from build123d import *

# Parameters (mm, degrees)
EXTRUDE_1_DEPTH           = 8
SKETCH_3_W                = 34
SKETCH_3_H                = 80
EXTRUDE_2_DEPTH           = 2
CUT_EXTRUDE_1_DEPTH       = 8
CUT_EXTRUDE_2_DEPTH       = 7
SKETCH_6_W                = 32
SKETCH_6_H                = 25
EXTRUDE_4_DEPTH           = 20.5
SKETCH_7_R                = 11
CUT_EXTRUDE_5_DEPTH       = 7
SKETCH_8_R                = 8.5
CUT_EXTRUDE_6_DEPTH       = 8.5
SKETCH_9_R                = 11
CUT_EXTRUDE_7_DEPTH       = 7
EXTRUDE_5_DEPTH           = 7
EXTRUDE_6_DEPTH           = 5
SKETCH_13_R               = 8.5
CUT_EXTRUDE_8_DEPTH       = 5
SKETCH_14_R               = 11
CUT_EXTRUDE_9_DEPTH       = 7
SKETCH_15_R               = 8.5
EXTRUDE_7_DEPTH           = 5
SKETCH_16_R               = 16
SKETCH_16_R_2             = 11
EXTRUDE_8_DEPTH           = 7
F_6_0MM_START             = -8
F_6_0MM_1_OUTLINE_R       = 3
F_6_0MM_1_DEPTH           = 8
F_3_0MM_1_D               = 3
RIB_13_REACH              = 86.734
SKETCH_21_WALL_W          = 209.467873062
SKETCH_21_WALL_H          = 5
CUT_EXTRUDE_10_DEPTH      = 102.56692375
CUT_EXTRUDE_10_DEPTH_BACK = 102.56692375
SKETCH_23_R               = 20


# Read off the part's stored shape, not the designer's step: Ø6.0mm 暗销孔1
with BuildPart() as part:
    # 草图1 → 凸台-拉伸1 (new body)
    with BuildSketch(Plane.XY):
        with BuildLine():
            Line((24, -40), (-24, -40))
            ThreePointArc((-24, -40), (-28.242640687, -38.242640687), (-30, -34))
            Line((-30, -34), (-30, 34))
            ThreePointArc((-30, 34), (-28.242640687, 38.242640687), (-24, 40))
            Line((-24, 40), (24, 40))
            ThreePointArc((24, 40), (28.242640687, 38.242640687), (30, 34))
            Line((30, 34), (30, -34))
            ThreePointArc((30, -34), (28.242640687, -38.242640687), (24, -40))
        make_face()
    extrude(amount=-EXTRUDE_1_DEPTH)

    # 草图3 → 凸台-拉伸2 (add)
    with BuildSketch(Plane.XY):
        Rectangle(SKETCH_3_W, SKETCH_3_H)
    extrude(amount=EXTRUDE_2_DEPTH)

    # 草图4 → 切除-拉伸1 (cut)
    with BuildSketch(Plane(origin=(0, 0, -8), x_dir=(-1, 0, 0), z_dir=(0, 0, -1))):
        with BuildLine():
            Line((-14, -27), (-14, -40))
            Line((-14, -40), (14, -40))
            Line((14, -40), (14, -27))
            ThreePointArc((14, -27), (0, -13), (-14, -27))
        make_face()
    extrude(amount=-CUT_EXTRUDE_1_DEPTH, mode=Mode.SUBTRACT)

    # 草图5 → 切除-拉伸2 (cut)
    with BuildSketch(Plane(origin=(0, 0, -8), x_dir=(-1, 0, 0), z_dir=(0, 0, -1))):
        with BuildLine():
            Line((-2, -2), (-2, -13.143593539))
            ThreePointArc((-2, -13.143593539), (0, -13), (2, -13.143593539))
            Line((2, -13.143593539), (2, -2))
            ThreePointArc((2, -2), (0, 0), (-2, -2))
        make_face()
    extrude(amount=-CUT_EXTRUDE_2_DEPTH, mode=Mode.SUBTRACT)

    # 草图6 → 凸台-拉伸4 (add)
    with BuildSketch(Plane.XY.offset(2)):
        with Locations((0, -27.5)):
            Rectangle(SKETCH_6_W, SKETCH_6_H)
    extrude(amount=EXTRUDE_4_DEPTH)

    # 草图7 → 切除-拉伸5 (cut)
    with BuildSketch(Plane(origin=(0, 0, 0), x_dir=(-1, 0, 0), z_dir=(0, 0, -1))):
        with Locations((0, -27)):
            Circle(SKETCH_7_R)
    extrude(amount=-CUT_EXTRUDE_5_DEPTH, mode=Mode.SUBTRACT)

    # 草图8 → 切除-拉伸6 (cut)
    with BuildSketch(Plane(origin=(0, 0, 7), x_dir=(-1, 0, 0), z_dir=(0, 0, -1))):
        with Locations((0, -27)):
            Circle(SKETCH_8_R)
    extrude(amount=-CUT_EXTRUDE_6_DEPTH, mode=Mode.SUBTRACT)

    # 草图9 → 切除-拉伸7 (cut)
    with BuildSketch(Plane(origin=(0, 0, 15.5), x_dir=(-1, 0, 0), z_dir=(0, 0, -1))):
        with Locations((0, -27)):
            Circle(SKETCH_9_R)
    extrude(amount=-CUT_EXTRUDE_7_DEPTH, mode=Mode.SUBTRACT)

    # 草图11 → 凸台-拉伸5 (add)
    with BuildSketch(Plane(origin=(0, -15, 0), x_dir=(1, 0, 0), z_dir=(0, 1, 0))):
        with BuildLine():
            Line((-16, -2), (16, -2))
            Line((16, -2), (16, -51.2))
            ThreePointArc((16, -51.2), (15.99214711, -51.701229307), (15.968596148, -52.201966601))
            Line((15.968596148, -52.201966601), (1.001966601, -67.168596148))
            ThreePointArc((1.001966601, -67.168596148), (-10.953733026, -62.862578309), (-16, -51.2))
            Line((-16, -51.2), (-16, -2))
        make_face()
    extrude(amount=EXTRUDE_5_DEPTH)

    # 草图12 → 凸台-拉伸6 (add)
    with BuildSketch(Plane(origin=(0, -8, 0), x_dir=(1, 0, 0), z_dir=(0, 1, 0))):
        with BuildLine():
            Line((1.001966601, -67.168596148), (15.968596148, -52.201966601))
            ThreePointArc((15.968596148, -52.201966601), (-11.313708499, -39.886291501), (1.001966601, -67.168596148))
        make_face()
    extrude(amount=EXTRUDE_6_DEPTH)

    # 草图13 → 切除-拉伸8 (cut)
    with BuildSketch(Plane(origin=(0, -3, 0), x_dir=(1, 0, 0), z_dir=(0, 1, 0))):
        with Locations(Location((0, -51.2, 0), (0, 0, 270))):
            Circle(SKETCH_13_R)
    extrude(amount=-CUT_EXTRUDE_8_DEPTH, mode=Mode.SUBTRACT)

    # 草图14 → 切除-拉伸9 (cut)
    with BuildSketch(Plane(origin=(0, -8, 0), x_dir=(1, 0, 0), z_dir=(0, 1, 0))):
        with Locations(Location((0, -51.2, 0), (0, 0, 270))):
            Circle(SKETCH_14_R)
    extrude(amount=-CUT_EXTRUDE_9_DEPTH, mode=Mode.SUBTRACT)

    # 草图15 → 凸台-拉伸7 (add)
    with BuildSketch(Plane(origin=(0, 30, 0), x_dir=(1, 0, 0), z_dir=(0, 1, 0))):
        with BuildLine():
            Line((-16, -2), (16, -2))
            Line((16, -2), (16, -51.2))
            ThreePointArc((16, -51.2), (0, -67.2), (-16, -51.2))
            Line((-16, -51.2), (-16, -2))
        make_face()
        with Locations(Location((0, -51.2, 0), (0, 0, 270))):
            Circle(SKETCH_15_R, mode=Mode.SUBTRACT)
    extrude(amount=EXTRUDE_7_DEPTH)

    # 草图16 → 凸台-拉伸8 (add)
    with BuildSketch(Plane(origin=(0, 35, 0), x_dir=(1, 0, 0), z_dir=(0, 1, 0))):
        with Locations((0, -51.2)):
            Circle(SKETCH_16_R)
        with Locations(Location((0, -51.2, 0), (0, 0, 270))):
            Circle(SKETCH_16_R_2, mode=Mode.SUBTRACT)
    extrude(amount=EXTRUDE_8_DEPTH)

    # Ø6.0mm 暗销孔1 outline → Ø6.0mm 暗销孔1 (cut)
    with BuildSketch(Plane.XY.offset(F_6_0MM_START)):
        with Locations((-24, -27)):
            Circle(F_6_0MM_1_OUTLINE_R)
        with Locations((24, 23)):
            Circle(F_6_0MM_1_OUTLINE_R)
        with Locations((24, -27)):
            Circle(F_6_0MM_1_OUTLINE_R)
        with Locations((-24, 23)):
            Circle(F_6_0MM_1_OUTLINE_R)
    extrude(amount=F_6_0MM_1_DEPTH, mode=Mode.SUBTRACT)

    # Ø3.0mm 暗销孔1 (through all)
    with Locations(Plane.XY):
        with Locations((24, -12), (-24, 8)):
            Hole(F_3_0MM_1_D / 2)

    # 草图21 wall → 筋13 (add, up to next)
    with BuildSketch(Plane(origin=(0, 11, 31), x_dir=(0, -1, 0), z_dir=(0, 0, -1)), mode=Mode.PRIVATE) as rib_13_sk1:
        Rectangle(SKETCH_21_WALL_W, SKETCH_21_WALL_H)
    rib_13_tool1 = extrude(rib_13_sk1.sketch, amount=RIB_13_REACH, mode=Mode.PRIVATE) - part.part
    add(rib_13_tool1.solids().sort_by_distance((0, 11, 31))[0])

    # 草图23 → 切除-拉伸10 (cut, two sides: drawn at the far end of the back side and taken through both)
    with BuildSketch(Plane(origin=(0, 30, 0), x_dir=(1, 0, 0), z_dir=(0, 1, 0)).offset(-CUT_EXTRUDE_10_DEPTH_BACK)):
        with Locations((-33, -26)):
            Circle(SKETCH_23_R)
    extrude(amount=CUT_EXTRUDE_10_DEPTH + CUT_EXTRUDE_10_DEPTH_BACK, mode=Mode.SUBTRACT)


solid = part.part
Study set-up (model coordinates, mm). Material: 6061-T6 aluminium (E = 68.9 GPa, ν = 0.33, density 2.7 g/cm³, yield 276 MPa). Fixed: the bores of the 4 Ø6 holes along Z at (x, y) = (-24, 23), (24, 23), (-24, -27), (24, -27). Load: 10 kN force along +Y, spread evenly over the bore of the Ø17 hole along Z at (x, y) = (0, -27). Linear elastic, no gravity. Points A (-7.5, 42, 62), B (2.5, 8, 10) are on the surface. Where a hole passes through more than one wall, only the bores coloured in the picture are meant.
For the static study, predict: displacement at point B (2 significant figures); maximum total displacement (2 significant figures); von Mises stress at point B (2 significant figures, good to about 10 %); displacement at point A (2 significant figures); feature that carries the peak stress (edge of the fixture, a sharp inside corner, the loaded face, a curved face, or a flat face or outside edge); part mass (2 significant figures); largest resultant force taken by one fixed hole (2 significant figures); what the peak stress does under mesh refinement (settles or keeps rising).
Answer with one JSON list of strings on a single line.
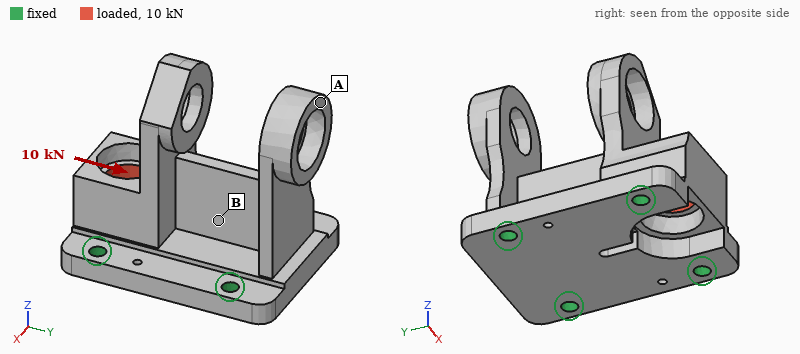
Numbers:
["15 µm", "56 µm", "26 MPa", "34 µm", "edge of the fixture", "200 g", "3.2 kN", "keeps rising"]
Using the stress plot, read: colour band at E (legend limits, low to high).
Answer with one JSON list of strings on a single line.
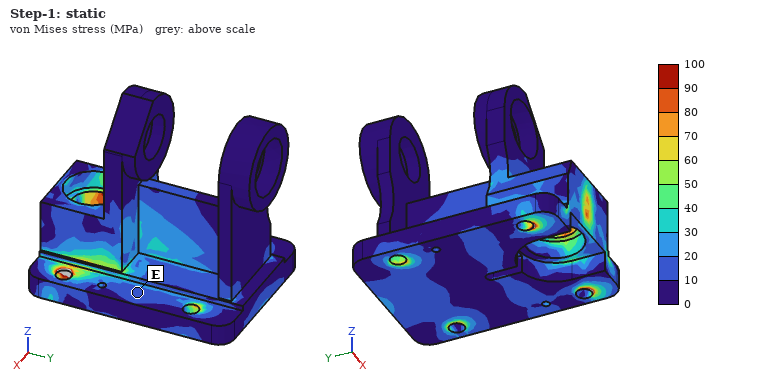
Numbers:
["10 to 20 MPa"]
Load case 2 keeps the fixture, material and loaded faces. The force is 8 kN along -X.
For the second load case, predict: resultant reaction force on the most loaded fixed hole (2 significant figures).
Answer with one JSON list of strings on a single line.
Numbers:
["4.2 kN"]
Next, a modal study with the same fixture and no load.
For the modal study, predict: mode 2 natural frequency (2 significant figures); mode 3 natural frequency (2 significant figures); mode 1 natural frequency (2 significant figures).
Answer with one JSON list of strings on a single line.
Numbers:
["3400 Hz", "3400 Hz", "2100 Hz"]
